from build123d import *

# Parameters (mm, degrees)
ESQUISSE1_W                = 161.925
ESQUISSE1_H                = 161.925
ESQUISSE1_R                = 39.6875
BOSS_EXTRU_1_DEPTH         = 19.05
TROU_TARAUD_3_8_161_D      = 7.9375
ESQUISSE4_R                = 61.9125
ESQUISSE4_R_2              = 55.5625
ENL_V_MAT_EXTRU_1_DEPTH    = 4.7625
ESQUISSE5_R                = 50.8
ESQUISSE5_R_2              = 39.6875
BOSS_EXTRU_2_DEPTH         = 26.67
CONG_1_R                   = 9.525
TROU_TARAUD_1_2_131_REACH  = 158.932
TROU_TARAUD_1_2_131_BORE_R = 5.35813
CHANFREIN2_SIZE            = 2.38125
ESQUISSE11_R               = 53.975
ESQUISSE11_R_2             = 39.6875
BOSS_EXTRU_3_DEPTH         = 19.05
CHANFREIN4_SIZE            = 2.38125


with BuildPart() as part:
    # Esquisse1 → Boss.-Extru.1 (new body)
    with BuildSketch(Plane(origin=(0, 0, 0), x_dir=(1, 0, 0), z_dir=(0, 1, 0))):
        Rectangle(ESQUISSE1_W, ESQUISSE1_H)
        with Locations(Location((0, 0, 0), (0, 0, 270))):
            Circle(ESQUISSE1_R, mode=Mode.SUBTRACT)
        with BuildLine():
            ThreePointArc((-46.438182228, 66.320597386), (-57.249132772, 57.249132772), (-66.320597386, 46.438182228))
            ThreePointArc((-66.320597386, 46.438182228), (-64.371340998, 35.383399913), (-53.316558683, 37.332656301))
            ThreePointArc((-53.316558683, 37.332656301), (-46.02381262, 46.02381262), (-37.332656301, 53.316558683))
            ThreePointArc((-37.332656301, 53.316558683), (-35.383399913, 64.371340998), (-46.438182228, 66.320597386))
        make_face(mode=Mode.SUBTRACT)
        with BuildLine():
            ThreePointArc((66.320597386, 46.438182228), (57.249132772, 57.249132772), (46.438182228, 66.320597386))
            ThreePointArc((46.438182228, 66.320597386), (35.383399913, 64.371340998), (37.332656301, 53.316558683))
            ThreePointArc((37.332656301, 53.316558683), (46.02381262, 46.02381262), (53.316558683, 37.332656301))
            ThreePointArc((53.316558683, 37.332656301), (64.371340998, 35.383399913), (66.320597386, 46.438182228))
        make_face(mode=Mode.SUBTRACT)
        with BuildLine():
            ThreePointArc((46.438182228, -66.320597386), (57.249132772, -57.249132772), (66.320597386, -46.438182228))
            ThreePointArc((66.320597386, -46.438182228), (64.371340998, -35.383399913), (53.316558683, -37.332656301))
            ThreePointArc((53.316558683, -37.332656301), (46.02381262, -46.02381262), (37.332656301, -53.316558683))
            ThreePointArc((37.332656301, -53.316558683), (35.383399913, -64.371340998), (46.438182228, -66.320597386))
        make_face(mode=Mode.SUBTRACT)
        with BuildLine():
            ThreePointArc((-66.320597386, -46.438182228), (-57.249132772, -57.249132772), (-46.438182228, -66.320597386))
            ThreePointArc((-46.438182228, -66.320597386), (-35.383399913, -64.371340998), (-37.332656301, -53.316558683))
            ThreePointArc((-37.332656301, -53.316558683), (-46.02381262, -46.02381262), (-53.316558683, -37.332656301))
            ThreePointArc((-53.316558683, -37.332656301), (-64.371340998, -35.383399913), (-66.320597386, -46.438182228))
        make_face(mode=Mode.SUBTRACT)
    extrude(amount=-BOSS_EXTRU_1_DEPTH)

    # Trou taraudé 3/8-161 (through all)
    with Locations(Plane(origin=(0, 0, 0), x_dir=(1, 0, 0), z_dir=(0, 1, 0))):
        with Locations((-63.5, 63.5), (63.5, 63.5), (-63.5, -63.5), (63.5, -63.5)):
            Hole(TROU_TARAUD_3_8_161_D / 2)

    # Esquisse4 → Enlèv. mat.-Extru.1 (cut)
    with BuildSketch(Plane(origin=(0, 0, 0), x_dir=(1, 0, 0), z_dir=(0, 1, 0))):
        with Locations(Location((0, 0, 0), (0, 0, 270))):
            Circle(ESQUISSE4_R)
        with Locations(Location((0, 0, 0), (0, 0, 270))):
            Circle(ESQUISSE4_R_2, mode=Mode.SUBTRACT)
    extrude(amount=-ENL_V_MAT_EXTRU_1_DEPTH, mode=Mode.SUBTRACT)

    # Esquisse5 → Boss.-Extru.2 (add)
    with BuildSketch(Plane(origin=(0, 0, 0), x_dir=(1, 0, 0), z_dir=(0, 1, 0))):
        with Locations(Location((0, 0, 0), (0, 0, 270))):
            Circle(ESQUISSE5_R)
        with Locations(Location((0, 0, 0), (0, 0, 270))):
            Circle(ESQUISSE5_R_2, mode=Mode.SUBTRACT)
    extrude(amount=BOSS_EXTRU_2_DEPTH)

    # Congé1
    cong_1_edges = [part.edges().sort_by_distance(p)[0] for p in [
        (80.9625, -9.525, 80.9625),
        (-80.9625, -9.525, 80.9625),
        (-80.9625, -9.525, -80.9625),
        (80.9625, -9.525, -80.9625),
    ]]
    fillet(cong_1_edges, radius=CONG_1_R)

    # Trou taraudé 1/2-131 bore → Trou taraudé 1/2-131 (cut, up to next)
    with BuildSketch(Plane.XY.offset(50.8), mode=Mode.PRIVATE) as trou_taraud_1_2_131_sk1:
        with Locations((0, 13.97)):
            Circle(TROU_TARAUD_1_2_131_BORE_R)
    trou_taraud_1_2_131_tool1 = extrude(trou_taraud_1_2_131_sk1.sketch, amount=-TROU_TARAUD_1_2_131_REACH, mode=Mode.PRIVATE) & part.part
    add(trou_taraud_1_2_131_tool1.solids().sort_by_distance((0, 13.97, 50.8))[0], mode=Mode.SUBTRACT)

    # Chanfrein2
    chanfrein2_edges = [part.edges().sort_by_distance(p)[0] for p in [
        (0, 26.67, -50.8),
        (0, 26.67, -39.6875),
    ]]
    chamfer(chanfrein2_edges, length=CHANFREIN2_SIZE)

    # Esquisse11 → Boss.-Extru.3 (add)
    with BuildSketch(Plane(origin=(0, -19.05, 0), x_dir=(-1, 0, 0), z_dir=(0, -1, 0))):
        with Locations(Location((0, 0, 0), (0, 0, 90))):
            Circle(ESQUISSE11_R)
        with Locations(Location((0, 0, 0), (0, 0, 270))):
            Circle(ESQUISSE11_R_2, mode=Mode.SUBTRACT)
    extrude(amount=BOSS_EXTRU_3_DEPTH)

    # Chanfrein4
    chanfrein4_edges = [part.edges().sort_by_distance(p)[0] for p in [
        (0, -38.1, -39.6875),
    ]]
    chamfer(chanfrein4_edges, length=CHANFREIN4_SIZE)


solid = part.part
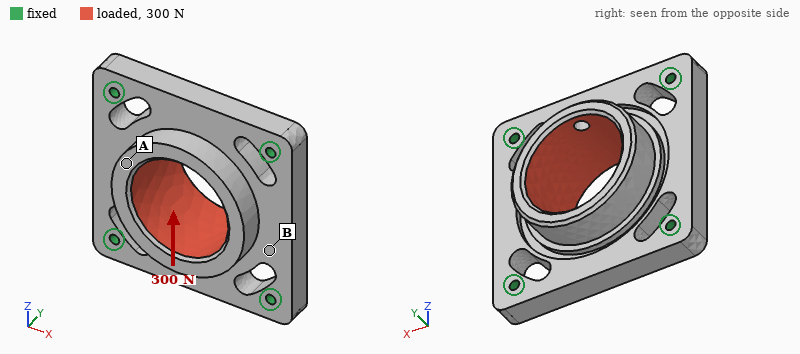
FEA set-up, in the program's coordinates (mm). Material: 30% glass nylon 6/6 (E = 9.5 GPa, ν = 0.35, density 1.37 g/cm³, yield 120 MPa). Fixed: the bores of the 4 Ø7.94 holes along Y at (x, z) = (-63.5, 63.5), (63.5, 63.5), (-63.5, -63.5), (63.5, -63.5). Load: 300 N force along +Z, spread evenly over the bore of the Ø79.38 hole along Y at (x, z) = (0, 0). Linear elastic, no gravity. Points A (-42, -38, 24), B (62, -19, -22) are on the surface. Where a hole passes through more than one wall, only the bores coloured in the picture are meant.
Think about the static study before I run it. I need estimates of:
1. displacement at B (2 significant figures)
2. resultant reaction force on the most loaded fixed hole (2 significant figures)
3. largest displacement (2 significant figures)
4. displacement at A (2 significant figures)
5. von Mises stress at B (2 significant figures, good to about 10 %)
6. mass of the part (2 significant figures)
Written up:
1.3 µm
75 N
3.1 µm
1.8 µm
0.15 MPa
690 g
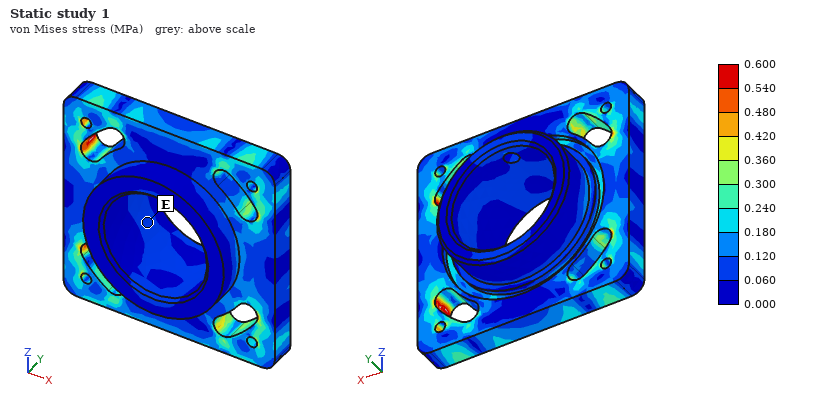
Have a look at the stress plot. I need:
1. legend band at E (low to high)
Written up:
0.060 to 0.120 MPa
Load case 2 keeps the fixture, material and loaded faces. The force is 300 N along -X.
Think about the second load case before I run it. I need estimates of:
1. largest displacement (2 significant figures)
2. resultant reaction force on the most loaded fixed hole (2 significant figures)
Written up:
3.0 µm
76 N
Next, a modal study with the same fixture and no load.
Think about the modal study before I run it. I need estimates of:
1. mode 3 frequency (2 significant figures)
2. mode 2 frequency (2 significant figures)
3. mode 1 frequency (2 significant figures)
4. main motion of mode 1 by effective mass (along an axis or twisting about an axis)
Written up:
1900 Hz
1900 Hz
1400 Hz
along Y
